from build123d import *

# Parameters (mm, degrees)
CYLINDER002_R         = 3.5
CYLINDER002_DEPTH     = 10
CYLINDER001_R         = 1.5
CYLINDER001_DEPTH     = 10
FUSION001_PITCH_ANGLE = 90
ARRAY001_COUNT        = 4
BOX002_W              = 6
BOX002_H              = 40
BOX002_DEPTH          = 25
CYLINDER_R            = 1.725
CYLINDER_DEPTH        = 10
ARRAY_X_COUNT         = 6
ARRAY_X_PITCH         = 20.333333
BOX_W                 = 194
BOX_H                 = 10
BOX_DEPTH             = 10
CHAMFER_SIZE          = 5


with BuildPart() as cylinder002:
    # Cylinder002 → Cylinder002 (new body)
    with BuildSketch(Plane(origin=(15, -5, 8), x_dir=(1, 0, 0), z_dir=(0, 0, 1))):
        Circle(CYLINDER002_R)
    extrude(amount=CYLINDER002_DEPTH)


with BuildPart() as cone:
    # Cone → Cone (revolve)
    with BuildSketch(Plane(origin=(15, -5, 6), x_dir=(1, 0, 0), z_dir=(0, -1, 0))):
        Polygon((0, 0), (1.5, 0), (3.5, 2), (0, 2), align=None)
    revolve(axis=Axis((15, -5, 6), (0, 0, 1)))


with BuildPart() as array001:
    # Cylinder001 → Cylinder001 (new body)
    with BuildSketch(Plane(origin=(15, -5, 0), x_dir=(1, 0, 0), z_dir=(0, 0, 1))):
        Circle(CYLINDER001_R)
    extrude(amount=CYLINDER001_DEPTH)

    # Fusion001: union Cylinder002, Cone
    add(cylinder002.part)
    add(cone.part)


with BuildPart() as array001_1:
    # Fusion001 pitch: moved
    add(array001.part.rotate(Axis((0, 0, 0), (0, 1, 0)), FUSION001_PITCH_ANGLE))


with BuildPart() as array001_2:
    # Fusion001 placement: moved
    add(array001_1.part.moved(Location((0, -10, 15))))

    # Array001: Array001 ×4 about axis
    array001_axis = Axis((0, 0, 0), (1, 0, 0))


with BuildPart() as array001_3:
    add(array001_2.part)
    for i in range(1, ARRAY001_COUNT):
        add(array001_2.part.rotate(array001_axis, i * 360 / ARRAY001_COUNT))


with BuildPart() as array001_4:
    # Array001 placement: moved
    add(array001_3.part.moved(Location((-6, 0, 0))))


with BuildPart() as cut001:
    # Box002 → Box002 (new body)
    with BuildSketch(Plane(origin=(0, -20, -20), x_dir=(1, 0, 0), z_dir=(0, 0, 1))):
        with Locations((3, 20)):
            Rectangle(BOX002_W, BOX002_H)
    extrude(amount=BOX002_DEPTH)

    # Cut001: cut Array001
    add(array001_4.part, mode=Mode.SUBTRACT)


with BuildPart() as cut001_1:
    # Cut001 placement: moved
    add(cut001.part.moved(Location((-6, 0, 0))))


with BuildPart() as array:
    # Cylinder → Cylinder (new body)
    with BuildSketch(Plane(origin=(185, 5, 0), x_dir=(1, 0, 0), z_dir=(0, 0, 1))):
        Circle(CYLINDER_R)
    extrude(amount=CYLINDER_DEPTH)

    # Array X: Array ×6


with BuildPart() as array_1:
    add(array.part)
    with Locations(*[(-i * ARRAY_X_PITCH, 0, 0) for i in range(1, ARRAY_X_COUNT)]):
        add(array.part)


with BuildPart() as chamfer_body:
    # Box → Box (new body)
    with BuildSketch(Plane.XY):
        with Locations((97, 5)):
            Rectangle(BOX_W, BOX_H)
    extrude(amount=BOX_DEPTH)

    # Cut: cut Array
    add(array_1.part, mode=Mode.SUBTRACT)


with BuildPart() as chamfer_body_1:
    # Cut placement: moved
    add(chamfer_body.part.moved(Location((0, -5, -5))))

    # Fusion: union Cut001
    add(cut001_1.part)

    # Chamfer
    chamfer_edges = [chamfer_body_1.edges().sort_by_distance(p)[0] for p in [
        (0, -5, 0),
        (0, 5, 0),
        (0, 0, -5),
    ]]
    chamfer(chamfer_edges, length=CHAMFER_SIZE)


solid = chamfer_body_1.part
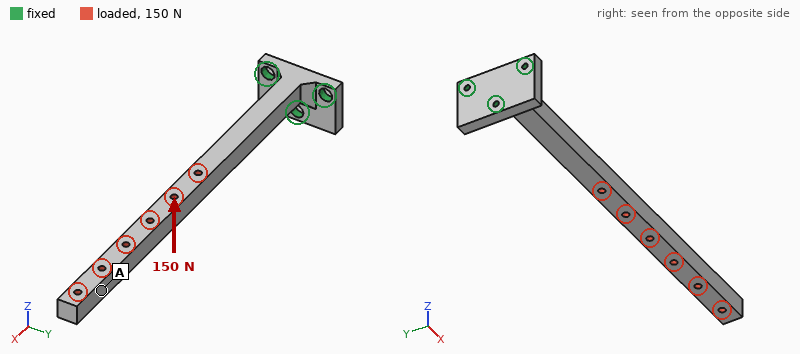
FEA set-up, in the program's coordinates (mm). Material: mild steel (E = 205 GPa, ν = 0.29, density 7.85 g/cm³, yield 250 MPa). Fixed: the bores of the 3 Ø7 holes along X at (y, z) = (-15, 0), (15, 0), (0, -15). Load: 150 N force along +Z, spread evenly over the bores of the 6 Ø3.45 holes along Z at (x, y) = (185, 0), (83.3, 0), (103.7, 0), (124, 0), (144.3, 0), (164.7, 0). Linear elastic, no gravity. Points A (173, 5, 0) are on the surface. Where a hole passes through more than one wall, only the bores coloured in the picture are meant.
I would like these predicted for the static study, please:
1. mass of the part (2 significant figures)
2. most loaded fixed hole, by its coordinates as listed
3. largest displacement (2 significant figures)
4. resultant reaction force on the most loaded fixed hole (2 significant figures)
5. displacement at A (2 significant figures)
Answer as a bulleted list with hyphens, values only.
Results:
- 190 g
- (0, -15)
- 1.3 mm
- 1.2 kN
- 1.1 mm
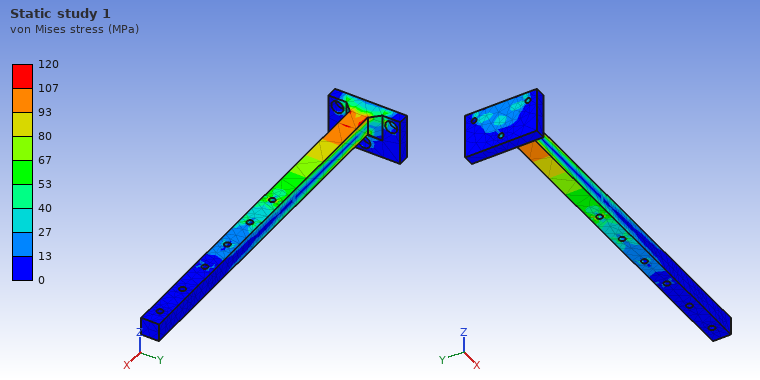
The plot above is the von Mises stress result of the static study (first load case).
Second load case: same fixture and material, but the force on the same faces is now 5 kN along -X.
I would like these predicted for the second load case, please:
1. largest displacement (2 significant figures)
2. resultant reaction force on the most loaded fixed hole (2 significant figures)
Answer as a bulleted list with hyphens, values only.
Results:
- 0.10 mm
- 2.3 kN
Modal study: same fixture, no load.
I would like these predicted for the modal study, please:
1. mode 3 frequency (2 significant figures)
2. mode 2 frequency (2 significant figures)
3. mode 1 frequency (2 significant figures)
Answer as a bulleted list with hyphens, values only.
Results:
- 1300 Hz
- 230 Hz
- 220 Hz
